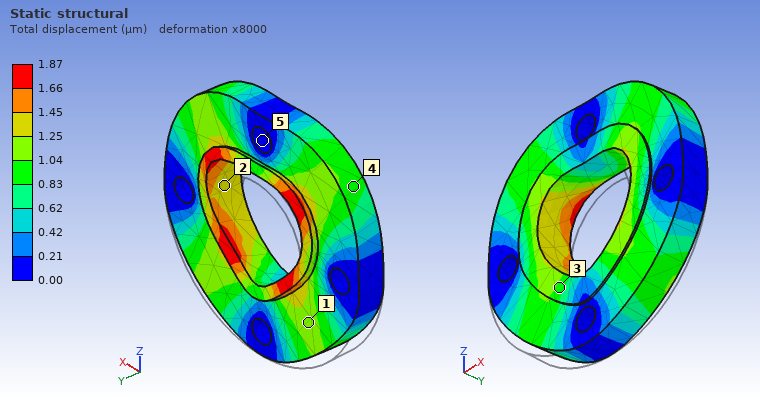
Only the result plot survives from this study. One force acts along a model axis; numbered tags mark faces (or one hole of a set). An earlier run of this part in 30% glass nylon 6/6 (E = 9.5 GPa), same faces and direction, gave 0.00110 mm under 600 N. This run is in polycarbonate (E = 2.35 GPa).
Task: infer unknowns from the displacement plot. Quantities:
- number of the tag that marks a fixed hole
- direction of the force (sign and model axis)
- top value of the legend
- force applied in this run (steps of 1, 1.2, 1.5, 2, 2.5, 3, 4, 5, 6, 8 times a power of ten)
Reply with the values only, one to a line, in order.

5
+Z
1.87 µm
250 N
